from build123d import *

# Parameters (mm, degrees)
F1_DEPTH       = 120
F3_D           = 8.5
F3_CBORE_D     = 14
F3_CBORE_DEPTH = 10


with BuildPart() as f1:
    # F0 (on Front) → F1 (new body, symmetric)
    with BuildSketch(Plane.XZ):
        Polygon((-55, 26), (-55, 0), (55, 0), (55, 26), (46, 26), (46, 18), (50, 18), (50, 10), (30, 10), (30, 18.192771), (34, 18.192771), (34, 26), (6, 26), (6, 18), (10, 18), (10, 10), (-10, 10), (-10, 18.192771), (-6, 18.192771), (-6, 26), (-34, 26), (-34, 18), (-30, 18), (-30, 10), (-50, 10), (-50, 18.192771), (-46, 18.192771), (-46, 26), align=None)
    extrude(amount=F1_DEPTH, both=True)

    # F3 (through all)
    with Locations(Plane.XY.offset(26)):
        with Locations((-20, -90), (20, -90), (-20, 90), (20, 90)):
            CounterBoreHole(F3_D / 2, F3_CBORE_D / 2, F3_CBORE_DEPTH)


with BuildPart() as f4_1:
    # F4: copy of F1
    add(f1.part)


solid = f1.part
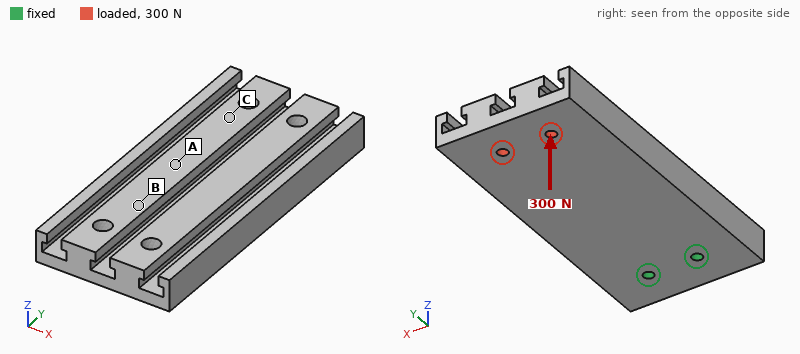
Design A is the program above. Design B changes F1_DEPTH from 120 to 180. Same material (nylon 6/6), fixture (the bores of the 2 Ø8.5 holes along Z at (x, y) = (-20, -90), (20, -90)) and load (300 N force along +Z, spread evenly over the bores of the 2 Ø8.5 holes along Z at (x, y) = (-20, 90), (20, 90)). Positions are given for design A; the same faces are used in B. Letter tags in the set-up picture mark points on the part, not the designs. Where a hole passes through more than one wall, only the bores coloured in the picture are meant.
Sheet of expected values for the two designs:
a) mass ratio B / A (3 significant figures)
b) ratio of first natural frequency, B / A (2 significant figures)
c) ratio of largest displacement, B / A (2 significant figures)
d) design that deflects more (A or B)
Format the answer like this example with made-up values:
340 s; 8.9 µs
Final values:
1.51; 0.63; 1.3; B
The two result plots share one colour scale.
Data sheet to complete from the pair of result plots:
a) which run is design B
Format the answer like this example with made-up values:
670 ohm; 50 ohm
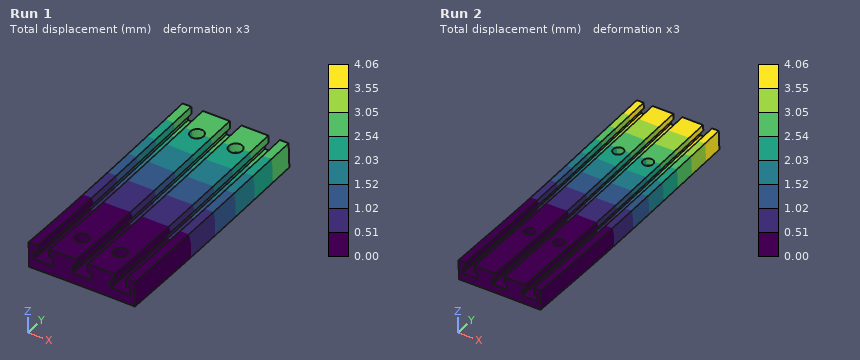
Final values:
Run 2
